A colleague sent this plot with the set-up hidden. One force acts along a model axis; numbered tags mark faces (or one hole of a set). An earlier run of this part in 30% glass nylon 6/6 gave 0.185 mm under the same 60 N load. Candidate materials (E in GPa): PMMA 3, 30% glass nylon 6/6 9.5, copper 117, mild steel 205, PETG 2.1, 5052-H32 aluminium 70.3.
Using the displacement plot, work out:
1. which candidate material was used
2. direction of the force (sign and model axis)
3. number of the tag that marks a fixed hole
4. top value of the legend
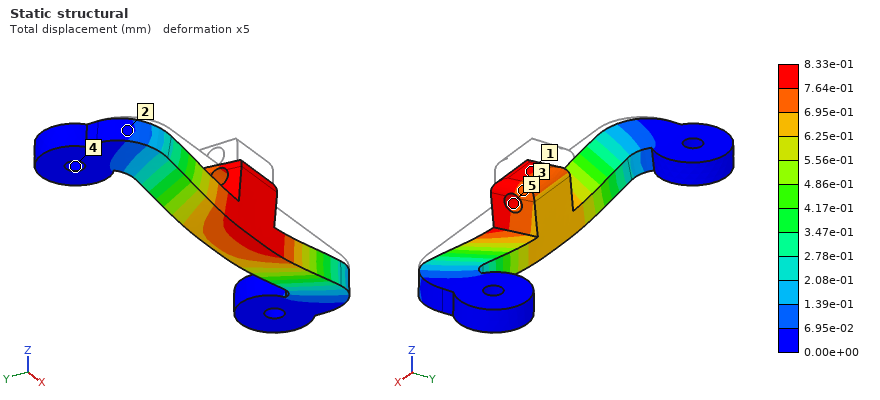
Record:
PETG
-Z
4
8.33e-01 mm
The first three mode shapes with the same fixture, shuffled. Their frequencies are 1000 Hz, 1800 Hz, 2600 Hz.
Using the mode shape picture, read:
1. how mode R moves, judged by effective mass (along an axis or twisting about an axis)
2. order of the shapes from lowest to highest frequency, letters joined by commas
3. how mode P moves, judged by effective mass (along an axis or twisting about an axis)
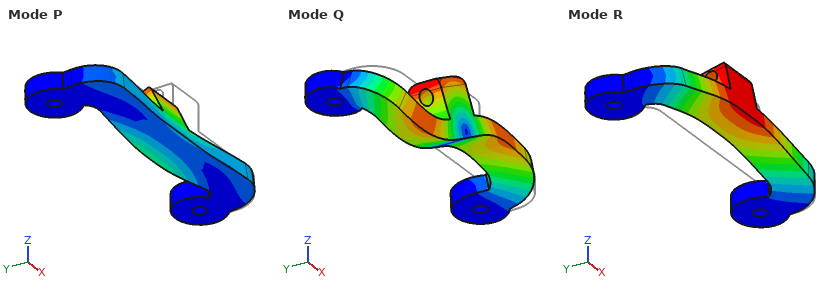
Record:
along Z
R, P, Q
along Y
